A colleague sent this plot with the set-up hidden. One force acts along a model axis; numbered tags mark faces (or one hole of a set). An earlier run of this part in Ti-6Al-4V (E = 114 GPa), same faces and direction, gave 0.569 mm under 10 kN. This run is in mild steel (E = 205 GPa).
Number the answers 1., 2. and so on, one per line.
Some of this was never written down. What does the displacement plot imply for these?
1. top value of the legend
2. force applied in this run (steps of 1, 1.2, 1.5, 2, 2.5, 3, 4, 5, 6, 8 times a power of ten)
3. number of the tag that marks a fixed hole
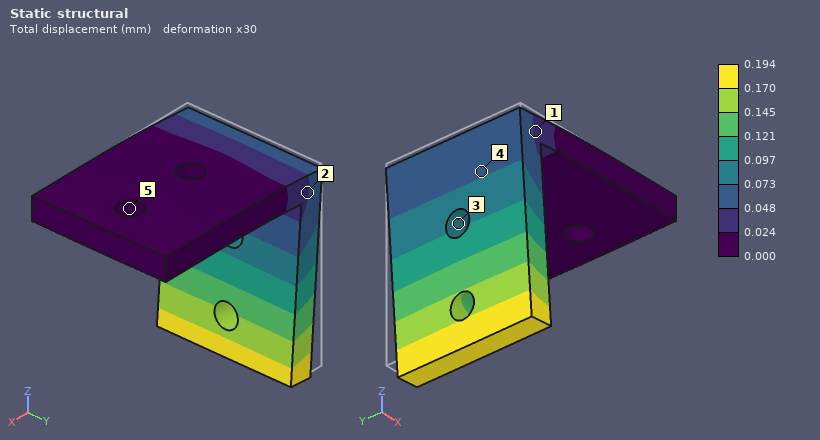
1. 0.194 mm
2. 6 kN
3. 5
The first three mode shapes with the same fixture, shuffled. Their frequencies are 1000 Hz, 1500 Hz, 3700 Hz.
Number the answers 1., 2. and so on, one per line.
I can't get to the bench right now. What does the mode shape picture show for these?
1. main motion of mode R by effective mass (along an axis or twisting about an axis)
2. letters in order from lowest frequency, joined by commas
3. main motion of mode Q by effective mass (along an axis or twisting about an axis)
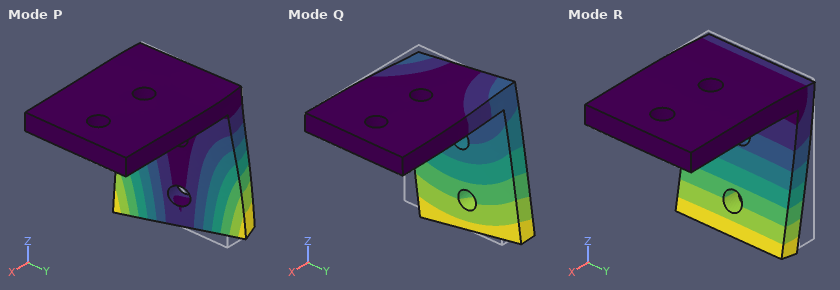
1. along X
2. R, Q, P
3. along Y
